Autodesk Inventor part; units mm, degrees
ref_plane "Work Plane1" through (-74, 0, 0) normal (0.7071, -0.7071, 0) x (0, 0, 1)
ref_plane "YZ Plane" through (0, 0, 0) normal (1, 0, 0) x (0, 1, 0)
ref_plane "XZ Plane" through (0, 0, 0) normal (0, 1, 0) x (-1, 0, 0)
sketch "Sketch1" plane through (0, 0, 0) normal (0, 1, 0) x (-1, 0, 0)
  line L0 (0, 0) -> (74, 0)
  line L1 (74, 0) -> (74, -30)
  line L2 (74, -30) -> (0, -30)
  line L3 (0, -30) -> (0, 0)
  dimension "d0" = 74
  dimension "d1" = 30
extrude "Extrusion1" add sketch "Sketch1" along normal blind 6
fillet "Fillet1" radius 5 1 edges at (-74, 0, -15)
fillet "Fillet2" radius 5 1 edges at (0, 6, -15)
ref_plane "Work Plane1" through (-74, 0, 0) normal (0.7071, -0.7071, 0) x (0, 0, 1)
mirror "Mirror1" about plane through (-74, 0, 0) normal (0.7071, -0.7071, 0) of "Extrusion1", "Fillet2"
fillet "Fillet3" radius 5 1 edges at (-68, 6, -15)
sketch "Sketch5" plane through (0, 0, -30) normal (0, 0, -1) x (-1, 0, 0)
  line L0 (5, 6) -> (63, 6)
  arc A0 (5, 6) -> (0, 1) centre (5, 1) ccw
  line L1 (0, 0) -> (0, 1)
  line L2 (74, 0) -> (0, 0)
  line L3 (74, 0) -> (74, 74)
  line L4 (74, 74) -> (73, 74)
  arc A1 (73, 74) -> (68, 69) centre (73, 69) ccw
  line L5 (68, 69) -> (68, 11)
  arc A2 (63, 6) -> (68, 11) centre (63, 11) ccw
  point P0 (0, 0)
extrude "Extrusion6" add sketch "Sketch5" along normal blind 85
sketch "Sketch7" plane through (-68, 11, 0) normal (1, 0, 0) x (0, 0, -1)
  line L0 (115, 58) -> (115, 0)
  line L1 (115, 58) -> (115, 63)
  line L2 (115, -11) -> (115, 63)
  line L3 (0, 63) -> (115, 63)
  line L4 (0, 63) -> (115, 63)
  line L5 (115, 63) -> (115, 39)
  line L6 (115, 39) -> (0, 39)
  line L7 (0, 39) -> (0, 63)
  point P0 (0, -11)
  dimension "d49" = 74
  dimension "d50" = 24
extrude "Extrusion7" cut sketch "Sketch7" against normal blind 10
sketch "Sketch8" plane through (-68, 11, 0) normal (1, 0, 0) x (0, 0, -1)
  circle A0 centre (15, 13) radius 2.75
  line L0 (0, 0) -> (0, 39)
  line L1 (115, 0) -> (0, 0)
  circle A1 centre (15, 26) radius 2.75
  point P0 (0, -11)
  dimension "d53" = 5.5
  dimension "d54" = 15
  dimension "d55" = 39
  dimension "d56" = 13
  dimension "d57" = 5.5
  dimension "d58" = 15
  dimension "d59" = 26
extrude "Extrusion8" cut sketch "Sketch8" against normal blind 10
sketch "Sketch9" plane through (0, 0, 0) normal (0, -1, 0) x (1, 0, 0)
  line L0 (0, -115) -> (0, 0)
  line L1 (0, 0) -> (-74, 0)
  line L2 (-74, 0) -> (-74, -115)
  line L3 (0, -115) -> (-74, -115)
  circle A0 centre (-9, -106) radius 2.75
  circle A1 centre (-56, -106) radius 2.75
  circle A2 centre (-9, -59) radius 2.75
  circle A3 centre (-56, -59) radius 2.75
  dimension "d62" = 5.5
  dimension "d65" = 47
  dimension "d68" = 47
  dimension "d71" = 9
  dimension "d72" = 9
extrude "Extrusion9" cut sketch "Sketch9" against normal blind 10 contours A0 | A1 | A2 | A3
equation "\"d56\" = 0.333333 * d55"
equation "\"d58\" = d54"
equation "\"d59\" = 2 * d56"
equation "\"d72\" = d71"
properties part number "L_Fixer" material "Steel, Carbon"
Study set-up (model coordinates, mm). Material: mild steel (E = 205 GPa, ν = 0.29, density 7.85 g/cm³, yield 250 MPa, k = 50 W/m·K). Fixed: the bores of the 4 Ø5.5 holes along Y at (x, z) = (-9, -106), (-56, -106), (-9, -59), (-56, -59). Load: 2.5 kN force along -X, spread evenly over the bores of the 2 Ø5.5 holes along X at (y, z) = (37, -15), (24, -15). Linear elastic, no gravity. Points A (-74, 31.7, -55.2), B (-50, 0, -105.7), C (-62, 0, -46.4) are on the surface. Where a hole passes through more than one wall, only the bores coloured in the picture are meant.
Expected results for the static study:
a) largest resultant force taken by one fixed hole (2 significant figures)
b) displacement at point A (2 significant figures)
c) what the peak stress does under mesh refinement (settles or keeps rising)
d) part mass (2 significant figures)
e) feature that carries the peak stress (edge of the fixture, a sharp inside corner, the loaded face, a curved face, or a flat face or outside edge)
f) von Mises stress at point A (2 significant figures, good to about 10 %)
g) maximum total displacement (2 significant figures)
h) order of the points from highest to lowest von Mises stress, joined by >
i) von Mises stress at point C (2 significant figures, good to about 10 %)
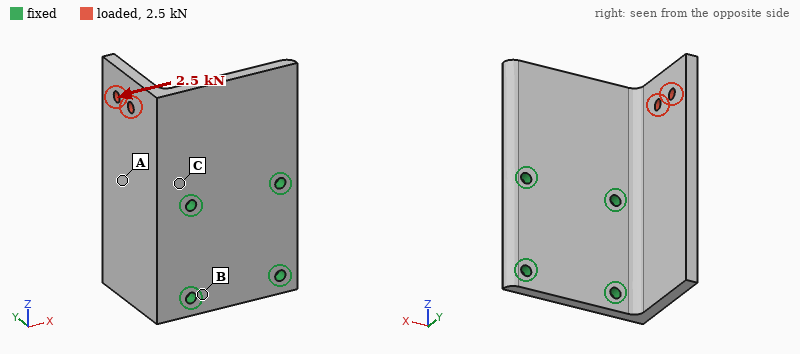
2.4 kN
0.12 mm
keeps rising
630 g
edge of the fixture
70 MPa
0.40 mm
C > A > B
110 MPa
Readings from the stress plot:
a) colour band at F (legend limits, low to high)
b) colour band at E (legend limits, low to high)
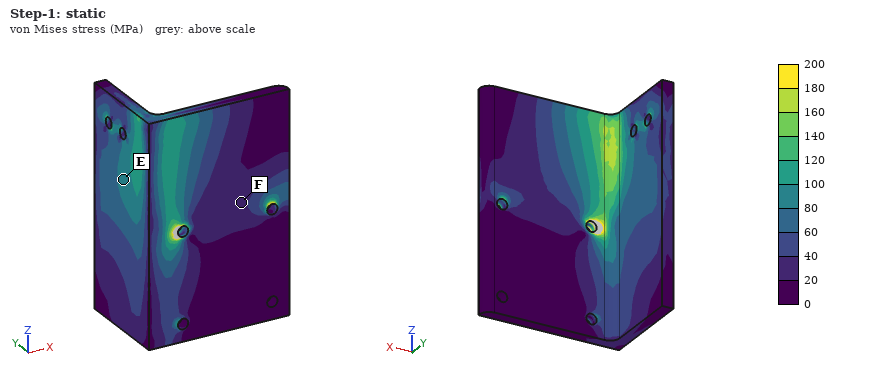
20 to 40 MPa
80 to 100 MPa
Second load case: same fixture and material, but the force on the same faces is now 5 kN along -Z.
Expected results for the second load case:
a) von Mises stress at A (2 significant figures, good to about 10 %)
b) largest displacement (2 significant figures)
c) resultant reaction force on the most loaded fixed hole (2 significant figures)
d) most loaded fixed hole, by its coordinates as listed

29 MPa
92 µm
4.2 kN
(-56, -59)
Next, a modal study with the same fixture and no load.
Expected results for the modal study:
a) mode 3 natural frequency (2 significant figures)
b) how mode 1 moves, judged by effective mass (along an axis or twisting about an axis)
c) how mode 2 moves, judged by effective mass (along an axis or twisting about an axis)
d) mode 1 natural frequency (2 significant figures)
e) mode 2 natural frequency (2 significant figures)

2300 Hz
along X
along Y
1400 Hz
2000 Hz
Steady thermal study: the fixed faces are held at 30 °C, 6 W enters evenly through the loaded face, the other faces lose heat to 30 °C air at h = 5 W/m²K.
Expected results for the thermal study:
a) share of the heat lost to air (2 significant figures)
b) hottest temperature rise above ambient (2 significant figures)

12 %
20 K
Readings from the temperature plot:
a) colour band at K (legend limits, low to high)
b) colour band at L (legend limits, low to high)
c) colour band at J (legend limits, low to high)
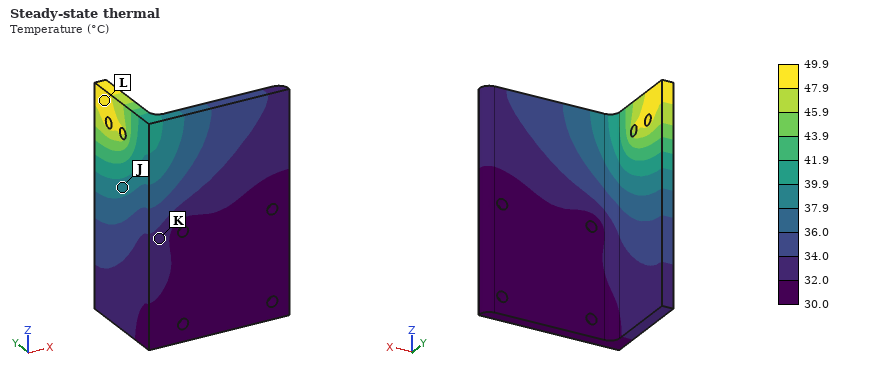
32.0 to 34.0 °C
47.9 to 49.9 °C
37.9 to 39.9 °C
